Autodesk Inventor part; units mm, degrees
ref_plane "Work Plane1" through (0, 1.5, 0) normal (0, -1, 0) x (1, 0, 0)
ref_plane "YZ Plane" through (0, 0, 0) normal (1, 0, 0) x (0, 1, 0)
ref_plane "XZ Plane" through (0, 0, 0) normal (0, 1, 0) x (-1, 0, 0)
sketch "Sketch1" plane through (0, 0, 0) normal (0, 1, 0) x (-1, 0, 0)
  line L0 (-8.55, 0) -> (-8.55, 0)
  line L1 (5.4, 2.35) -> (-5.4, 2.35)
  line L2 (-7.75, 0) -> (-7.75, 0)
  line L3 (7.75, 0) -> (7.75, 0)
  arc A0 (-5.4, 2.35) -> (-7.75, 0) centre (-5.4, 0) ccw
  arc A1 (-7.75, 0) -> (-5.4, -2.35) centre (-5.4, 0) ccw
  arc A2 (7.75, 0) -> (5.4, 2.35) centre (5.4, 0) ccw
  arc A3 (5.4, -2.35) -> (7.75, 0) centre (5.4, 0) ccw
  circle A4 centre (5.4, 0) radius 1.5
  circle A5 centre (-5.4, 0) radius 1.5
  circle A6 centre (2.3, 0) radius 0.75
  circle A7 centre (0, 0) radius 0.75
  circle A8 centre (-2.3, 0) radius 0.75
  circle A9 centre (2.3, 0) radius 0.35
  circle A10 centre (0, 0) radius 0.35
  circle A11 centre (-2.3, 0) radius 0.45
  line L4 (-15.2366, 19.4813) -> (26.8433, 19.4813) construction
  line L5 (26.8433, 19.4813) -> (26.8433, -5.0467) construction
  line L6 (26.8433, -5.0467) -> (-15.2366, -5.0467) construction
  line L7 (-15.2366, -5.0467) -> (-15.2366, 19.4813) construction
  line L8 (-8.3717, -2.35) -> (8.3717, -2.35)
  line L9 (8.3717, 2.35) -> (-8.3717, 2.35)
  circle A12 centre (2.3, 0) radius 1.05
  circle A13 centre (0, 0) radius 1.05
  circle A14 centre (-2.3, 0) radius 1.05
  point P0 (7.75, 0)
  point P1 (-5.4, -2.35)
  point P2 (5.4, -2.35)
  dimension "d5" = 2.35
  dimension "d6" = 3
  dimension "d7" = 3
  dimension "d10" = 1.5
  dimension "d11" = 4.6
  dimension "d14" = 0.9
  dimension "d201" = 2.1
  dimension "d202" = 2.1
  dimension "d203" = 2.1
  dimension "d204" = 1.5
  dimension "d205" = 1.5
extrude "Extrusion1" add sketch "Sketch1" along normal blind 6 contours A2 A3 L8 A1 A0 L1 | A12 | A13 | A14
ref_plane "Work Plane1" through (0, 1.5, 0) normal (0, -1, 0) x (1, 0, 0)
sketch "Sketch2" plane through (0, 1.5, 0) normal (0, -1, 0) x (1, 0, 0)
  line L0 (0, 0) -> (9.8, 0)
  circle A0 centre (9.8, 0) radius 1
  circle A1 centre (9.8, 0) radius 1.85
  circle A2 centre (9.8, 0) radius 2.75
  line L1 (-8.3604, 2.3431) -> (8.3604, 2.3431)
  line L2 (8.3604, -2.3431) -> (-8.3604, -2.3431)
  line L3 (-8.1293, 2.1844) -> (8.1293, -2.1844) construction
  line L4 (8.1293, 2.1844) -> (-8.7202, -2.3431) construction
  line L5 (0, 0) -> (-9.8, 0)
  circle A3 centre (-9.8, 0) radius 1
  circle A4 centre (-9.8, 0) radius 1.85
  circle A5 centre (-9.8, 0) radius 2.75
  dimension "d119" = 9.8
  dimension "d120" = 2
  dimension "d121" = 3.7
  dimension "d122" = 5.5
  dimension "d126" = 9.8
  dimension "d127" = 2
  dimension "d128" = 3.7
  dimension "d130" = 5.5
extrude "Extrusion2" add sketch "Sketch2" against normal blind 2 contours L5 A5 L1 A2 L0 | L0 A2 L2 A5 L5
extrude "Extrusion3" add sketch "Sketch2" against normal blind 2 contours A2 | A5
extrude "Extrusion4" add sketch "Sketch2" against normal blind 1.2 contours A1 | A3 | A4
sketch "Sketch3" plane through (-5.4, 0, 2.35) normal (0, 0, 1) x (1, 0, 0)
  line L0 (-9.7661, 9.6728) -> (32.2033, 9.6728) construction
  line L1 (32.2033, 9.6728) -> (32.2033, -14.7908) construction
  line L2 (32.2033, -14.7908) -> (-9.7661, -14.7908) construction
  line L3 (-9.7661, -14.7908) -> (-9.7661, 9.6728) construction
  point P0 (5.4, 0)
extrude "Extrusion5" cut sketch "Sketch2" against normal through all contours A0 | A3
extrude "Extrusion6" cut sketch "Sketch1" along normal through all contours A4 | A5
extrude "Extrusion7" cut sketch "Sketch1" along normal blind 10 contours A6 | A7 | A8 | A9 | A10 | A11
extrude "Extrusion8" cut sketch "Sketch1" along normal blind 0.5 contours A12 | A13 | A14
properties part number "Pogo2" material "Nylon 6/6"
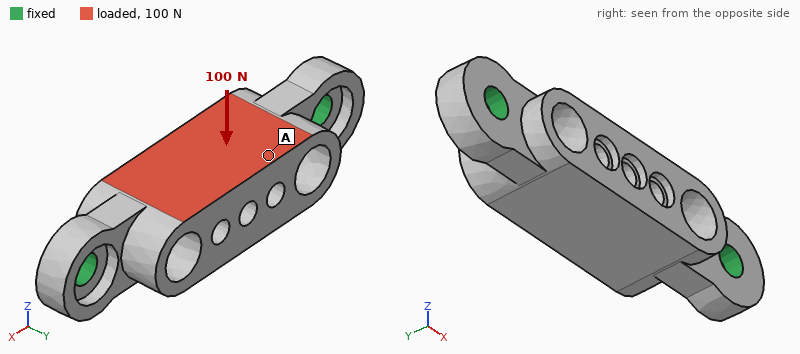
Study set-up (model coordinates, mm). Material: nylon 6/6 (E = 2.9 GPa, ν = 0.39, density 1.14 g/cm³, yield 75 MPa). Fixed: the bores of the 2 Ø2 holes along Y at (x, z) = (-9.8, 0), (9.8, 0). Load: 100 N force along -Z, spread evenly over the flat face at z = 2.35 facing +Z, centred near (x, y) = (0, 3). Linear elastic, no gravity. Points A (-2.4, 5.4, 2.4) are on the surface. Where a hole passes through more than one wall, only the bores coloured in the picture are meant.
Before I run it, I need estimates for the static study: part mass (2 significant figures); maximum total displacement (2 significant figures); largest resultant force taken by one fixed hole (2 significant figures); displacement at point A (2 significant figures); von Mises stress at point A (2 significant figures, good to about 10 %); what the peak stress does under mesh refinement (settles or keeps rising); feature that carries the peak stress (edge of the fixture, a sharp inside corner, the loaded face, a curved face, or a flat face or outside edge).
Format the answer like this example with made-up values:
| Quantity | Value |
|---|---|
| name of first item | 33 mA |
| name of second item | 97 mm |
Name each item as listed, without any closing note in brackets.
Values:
| Quantity | Value |
|---|---|
| part mass | 0.41 g |
| maximum total displacement | 0.18 mm |
| largest resultant force taken by one fixed hole | 50 N |
| displacement at point A | 0.16 mm |
| von Mises stress at point A | 10.0 MPa |
| what the peak stress does under mesh refinement | keeps rising |
| feature that carries the peak stress | edge of the fixture |
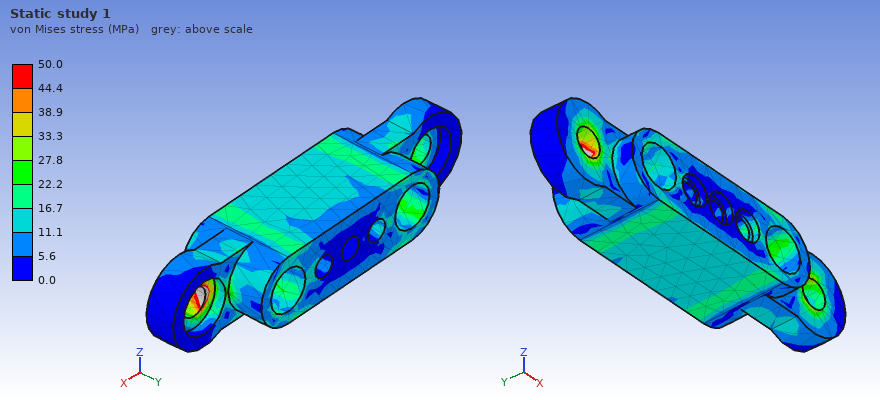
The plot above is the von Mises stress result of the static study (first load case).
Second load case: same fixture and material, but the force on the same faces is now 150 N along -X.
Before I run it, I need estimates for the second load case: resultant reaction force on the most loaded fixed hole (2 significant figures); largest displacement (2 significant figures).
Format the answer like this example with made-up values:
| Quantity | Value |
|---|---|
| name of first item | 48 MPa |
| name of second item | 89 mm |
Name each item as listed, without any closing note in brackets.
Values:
| Quantity | Value |
|---|---|
| resultant reaction force on the most loaded fixed hole | 78 N |
| largest displacement | 38 µm |
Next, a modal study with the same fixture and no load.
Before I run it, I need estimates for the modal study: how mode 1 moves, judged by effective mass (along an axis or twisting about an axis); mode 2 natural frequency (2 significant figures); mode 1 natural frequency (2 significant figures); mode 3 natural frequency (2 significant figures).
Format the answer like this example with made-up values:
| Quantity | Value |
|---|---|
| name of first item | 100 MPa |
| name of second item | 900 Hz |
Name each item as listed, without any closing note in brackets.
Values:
| Quantity | Value |
|---|---|
| how mode 1 moves, judged by effective mass | along Z |
| mode 2 natural frequency | 10000 Hz |
| mode 1 natural frequency | 7500 Hz |
| mode 3 natural frequency | 10000 Hz |
